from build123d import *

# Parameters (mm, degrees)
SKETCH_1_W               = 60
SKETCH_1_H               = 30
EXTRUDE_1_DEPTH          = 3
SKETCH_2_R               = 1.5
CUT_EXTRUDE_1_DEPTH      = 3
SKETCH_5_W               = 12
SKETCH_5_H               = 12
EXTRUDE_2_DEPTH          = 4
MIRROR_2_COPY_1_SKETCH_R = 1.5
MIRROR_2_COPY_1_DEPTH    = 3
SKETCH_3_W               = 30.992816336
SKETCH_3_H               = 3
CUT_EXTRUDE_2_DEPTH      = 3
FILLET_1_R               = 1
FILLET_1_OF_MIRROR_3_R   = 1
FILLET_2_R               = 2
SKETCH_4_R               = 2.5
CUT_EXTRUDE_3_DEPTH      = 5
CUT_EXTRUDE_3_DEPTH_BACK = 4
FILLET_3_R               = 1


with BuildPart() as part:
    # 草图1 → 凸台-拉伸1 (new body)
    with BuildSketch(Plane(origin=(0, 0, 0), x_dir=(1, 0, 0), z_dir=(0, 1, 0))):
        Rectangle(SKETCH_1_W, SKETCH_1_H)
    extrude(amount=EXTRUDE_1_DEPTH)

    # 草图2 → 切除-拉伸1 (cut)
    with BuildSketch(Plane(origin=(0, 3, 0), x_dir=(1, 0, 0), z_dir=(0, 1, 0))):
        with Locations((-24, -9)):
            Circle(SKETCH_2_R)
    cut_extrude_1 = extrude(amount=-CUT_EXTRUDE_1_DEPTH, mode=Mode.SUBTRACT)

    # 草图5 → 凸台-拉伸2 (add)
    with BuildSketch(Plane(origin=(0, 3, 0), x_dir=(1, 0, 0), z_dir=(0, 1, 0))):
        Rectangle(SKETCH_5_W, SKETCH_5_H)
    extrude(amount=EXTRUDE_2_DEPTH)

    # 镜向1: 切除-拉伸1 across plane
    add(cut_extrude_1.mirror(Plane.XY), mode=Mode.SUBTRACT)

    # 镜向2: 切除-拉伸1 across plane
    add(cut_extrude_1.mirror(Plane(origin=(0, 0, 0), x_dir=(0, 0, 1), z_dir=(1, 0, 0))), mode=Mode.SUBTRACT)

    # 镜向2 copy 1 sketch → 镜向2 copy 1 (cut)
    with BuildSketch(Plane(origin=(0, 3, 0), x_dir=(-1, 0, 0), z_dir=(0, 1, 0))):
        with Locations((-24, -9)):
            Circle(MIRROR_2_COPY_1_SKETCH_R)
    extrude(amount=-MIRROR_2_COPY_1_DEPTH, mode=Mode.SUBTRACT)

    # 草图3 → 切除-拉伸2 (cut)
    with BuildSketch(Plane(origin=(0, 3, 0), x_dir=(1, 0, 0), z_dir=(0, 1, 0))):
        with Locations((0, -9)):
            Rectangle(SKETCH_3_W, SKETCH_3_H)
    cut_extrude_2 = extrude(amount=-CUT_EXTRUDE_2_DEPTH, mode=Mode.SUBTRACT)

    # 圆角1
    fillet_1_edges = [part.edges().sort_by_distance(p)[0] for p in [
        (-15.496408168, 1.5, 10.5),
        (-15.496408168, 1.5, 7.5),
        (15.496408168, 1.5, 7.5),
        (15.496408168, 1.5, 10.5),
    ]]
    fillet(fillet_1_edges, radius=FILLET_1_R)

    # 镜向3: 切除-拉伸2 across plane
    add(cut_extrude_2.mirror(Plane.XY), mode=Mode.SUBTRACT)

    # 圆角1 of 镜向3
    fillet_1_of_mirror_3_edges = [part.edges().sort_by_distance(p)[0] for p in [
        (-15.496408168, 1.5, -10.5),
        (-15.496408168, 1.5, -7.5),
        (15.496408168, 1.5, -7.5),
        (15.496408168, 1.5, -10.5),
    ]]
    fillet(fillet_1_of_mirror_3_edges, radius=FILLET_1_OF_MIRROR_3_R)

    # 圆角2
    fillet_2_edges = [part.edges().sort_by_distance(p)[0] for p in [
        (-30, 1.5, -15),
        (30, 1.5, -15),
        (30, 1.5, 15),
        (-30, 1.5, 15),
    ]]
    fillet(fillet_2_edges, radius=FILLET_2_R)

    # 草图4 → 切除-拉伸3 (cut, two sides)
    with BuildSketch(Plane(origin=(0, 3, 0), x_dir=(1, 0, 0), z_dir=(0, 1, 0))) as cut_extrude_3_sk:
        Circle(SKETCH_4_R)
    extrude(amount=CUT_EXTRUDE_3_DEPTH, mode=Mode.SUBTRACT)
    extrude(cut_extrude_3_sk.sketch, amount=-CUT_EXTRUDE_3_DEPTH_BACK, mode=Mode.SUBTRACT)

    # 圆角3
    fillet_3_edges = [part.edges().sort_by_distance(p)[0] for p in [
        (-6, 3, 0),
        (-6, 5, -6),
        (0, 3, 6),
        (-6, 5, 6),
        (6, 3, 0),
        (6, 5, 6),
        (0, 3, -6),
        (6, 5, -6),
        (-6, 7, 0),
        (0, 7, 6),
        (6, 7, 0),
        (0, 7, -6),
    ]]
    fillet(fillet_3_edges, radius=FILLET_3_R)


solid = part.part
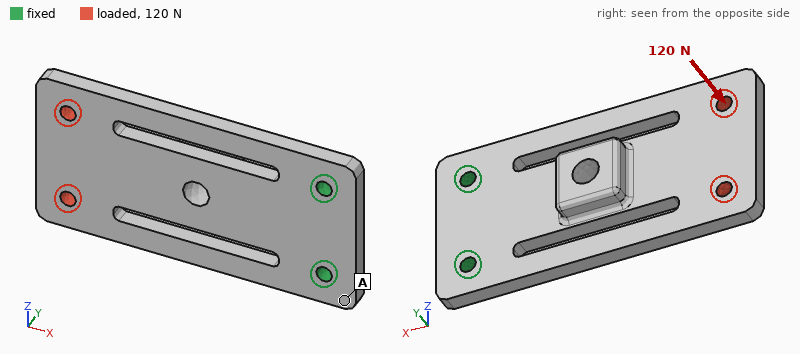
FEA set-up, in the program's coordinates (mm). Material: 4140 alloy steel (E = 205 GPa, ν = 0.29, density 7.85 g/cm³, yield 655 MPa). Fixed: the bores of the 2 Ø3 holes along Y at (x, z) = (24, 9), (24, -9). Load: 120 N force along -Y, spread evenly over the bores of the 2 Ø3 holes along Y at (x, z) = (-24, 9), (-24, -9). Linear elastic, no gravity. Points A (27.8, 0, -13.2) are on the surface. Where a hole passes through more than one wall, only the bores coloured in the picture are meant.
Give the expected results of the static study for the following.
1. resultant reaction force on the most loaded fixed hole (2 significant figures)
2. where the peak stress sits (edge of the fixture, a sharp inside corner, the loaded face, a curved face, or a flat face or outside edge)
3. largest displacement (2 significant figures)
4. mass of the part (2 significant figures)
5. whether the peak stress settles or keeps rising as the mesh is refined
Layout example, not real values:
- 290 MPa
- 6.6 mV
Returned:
- 62 N
- edge of the fixture
- 0.39 mm
- 41 g
- keeps rising
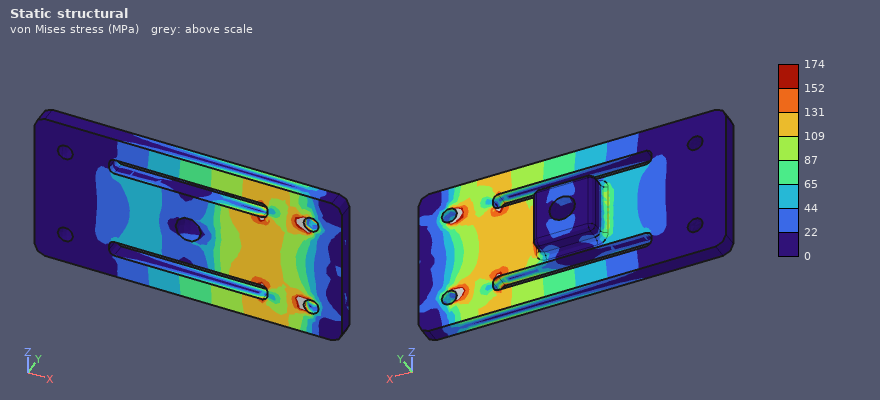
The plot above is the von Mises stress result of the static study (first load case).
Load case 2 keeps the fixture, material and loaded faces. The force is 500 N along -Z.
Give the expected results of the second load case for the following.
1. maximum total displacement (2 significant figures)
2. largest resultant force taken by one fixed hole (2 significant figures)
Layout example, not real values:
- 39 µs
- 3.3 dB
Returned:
- 37 µm
- 1.3 kN
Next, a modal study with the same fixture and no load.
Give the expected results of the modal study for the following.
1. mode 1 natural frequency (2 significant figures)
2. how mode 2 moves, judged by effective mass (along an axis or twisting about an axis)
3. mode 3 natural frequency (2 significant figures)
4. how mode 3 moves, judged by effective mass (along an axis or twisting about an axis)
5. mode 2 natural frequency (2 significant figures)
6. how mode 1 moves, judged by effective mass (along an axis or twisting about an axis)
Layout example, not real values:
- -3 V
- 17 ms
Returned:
- 850 Hz
- twisting about X
- 5100 Hz
- along Z
- 3300 Hz
- along Y
